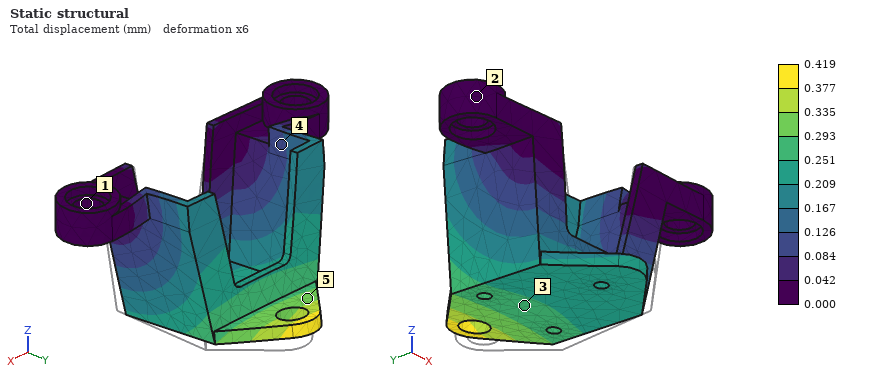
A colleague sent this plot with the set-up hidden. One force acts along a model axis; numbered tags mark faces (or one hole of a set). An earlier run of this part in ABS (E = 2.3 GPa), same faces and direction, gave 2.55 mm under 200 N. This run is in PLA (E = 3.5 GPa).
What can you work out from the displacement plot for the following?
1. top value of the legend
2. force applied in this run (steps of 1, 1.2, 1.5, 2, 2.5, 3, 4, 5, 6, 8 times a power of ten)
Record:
0.419 mm
50 N
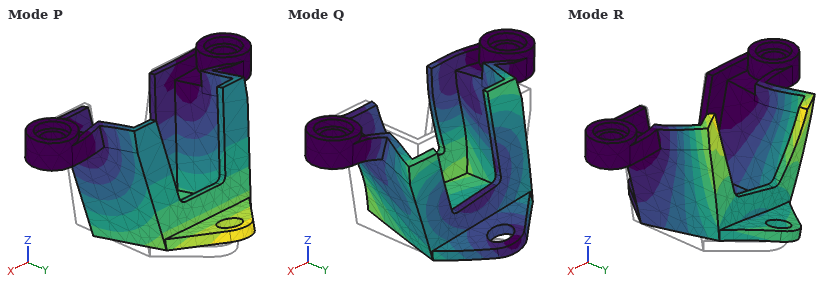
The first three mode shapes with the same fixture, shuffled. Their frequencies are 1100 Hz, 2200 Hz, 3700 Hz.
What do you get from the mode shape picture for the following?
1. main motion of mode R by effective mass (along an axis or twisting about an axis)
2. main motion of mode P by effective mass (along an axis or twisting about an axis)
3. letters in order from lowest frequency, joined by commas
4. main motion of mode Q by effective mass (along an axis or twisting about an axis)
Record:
along X
along Y
P, R, Q
along X
